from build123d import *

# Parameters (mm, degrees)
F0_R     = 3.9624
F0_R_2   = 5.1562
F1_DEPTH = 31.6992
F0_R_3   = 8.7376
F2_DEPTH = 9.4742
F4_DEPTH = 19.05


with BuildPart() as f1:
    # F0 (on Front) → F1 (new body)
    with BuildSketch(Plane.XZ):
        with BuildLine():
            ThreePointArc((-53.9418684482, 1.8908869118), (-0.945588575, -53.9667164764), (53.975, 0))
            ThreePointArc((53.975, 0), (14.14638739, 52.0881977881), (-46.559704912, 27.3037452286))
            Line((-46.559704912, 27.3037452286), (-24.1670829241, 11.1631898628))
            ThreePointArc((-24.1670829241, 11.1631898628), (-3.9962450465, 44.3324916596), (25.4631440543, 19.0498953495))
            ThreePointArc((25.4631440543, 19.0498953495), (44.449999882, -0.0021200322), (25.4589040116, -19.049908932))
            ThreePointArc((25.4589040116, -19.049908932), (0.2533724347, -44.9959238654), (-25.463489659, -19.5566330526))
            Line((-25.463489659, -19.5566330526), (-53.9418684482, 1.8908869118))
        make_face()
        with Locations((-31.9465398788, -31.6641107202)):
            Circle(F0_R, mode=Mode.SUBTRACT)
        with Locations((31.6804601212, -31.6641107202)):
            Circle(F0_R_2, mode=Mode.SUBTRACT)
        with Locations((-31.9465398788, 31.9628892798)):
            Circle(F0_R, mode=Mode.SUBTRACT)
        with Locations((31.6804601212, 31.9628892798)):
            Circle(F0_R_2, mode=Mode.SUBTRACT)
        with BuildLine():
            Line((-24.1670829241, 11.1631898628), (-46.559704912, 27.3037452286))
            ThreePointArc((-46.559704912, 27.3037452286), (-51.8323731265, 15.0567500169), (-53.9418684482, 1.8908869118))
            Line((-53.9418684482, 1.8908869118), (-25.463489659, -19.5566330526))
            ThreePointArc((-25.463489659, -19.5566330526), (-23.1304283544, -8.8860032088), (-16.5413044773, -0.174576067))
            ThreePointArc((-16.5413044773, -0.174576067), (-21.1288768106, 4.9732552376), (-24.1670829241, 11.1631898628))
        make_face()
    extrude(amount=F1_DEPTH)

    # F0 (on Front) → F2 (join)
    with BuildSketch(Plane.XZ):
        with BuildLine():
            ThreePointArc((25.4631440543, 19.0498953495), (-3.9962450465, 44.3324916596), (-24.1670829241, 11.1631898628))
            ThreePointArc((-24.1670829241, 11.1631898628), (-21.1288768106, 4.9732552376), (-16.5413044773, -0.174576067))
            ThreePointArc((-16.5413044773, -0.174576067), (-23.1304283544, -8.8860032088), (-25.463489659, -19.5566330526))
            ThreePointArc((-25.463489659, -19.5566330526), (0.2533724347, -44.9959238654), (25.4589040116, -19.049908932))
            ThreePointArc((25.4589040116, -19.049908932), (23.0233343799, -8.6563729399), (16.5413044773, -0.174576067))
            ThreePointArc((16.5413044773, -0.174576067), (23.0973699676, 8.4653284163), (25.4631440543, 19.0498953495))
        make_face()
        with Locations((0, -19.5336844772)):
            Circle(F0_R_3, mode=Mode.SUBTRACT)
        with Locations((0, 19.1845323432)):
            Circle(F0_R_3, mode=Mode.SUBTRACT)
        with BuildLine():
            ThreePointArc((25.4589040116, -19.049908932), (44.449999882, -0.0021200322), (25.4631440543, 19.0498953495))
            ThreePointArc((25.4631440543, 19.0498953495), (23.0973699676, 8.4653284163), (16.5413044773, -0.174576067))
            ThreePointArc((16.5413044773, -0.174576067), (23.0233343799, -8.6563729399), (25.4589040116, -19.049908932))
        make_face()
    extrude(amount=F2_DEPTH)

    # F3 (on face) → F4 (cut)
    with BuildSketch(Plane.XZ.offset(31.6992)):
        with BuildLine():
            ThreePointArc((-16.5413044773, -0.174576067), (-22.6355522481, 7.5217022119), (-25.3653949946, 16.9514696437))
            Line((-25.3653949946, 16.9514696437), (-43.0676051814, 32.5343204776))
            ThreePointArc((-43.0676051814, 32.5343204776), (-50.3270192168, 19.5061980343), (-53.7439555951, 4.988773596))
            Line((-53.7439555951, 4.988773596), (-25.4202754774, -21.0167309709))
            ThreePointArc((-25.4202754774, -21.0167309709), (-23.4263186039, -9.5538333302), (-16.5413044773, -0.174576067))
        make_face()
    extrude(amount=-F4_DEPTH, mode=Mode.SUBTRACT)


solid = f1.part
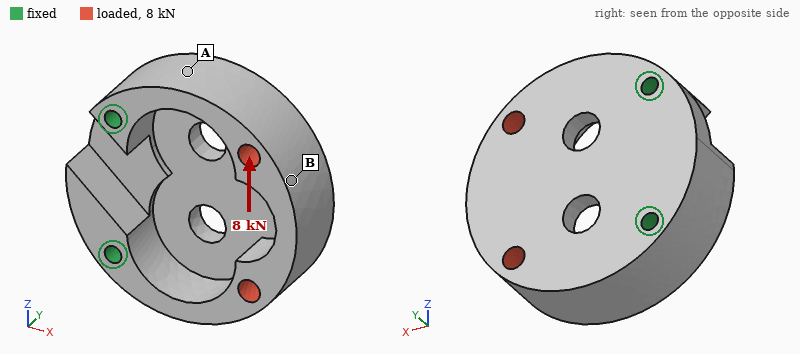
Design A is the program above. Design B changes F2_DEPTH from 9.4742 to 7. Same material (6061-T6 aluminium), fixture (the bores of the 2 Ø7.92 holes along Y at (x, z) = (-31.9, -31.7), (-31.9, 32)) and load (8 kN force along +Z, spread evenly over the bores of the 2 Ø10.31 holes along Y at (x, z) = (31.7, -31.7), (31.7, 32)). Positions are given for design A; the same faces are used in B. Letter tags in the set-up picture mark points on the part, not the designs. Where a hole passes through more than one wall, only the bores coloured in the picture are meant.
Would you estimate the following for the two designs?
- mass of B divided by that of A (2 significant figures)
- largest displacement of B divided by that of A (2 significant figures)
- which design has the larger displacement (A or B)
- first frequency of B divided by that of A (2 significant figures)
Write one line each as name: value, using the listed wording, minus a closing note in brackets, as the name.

mass of B divided by that of A: 0.94
largest displacement of B divided by that of A: 1.2
which design has the larger displacement: B
first frequency of B divided by that of A: 0.98
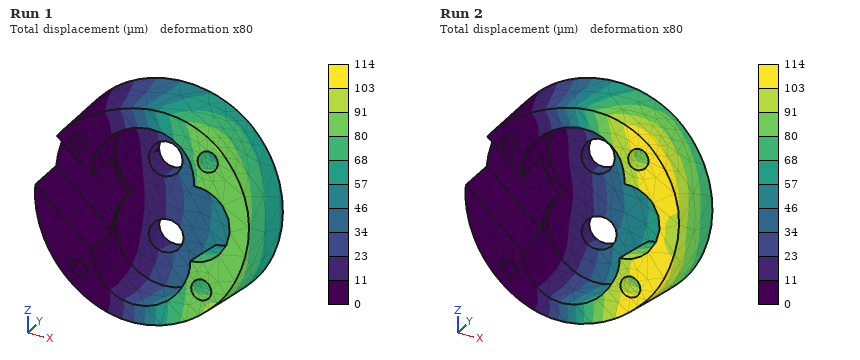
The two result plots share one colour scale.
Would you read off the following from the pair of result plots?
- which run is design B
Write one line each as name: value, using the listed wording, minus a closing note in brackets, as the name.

which run is design B: Run 2
